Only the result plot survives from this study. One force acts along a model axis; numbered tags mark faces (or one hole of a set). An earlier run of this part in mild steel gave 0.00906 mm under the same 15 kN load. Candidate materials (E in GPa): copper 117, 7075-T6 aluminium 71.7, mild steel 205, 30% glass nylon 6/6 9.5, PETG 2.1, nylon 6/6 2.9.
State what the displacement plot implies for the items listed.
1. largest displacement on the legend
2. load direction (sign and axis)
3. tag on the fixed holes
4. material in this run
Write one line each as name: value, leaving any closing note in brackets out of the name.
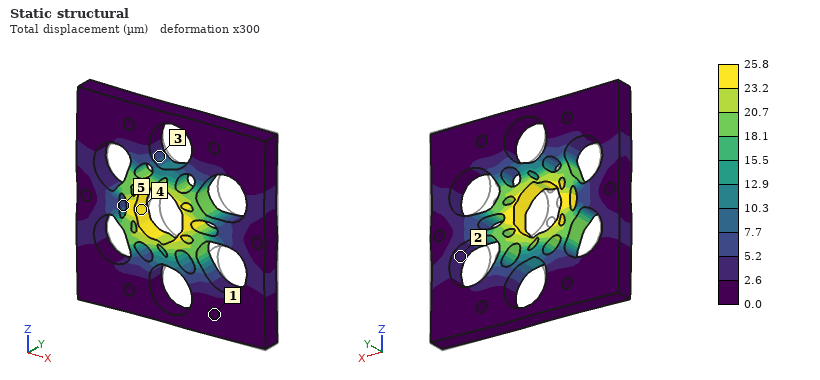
largest displacement on the legend: 25.8 µm
load direction: -X
tag on the fixed holes: 1
material in this run: 7075-T6 aluminium
